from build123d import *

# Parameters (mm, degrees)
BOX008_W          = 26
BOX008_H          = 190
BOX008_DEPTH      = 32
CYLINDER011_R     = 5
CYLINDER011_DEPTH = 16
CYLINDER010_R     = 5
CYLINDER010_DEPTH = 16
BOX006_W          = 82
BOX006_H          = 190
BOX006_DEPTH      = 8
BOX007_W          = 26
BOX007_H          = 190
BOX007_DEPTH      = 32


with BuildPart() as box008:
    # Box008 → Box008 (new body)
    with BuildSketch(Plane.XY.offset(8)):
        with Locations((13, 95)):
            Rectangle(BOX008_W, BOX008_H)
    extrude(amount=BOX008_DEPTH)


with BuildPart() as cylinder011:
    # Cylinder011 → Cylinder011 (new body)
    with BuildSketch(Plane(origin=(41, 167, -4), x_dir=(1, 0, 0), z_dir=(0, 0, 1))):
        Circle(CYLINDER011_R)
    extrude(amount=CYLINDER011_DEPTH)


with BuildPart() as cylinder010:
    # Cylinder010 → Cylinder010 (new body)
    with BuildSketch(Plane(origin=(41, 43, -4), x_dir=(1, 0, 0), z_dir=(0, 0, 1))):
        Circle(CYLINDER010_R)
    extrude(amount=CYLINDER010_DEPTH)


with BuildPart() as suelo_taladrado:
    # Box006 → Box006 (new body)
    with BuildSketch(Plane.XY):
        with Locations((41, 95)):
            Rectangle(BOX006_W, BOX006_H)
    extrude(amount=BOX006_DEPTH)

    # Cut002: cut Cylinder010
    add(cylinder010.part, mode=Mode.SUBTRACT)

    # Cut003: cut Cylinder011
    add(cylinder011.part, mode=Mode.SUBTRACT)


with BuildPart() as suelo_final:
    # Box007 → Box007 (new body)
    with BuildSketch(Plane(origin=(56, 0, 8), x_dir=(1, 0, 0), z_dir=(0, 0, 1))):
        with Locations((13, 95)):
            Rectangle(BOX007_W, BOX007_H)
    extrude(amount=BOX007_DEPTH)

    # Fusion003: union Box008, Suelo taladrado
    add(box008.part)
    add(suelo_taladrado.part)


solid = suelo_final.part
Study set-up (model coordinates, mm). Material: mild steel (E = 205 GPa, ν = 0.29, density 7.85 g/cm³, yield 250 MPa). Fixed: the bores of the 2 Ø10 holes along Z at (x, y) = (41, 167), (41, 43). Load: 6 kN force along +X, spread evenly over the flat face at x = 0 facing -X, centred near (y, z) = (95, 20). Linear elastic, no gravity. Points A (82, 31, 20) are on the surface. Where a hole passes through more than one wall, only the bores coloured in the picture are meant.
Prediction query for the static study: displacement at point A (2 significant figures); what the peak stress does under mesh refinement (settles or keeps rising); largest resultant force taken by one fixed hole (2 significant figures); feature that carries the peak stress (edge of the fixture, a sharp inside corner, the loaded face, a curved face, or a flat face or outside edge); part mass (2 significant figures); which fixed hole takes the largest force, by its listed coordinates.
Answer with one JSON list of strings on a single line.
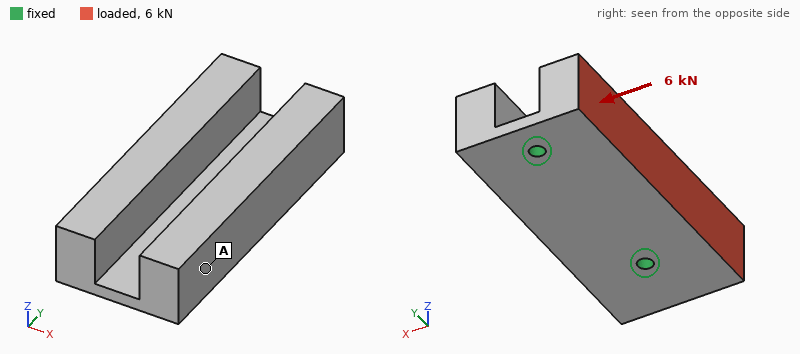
["16 µm", "keeps rising", "3.5 kN", "edge of the fixture", "3.5 kg", "(41, 43)"]
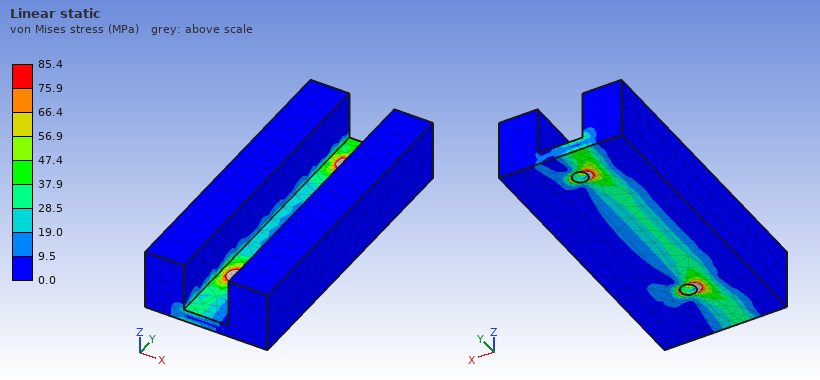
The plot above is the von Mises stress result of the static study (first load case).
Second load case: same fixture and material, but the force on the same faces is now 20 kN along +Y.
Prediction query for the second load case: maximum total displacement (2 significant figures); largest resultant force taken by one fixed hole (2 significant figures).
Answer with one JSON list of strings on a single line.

["20 µm", "13 kN"]
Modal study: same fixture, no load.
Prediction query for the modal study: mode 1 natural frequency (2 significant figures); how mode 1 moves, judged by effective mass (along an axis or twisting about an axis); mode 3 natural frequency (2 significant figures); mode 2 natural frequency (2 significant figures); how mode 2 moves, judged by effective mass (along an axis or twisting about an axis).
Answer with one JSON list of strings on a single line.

["1000 Hz", "along X", "2900 Hz", "1400 Hz", "along Z"]
